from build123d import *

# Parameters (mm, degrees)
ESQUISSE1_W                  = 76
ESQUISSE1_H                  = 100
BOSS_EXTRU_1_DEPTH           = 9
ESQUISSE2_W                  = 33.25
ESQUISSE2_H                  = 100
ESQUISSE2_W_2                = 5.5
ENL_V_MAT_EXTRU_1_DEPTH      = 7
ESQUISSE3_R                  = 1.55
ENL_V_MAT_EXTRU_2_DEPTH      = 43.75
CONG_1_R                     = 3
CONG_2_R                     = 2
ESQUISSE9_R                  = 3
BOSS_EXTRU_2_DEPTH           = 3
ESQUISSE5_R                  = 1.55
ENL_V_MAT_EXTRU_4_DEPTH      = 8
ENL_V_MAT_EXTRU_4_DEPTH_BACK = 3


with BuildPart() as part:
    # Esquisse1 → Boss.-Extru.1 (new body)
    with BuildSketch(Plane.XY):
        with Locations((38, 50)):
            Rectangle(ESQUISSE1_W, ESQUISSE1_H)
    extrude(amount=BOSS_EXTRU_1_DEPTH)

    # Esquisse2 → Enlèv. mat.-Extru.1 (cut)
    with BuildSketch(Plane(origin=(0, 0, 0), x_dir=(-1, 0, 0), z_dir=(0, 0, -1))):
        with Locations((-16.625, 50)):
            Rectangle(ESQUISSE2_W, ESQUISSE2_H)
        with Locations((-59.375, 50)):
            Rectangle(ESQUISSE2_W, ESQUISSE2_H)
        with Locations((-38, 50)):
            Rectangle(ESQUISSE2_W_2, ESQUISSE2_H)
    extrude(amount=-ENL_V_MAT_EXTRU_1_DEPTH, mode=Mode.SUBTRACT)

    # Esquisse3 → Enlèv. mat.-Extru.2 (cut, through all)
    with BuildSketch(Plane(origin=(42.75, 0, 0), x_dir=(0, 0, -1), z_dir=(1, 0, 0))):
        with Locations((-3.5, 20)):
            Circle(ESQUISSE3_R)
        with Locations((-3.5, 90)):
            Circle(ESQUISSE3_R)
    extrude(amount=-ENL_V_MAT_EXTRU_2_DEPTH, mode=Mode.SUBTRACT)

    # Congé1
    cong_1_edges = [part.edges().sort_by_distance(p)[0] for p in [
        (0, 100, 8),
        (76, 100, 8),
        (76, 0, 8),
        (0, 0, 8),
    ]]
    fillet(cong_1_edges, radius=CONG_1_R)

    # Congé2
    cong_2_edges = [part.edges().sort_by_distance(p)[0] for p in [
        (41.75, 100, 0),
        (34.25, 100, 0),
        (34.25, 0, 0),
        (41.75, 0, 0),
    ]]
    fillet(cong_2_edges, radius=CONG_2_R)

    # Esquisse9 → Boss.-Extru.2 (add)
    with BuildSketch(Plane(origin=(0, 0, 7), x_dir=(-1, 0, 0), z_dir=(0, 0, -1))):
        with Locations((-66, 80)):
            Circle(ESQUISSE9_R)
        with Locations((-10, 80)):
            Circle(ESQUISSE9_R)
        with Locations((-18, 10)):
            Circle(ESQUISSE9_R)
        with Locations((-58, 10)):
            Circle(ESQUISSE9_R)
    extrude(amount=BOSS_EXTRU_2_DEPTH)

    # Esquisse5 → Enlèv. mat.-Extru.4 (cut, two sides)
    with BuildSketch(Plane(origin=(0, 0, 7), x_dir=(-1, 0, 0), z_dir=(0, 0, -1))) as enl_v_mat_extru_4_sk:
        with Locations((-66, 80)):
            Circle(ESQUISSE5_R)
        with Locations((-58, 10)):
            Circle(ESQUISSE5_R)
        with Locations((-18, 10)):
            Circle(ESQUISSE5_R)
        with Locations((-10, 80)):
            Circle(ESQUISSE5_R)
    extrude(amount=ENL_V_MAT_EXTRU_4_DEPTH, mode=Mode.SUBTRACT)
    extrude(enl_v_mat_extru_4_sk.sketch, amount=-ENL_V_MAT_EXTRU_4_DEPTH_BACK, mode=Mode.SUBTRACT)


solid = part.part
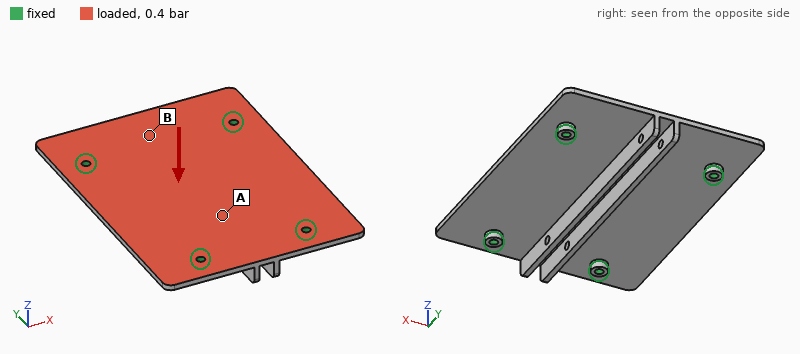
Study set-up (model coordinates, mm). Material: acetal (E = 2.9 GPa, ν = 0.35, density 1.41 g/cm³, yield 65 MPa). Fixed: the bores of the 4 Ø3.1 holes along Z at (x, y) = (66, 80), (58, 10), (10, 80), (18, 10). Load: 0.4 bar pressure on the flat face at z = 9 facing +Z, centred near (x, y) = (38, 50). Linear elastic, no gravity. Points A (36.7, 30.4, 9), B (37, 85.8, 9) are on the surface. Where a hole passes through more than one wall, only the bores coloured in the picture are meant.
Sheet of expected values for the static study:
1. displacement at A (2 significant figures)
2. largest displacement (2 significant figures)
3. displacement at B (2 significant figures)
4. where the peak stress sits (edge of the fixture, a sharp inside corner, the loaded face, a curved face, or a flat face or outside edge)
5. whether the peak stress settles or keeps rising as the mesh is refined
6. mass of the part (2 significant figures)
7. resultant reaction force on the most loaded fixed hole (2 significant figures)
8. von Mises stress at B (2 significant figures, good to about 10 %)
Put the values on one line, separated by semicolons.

0.56 mm; 1.2 mm; 0.84 mm; edge of the fixture; keeps rising; 26 g; 84 N; 12 MPa
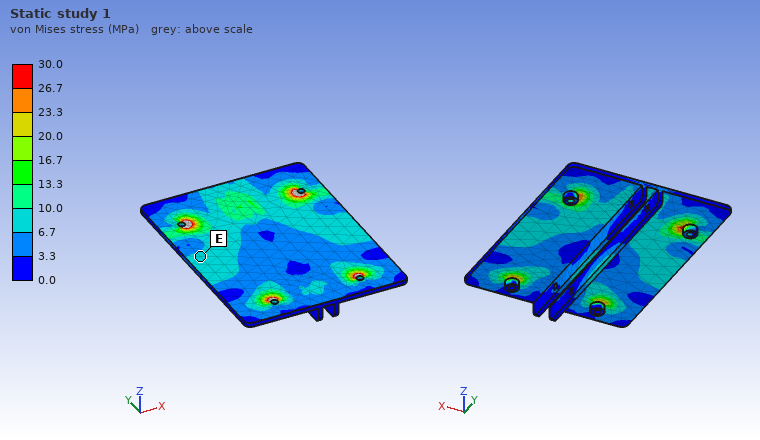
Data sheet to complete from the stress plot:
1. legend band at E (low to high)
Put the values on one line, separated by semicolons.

6.7 to 10.0 MPa
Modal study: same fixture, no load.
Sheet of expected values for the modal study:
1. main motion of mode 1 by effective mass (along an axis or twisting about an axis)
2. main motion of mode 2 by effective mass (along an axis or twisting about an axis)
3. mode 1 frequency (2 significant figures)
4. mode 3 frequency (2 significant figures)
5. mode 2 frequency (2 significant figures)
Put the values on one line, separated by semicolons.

along Z; twisting about Y; 620 Hz; 760 Hz; 690 Hz
